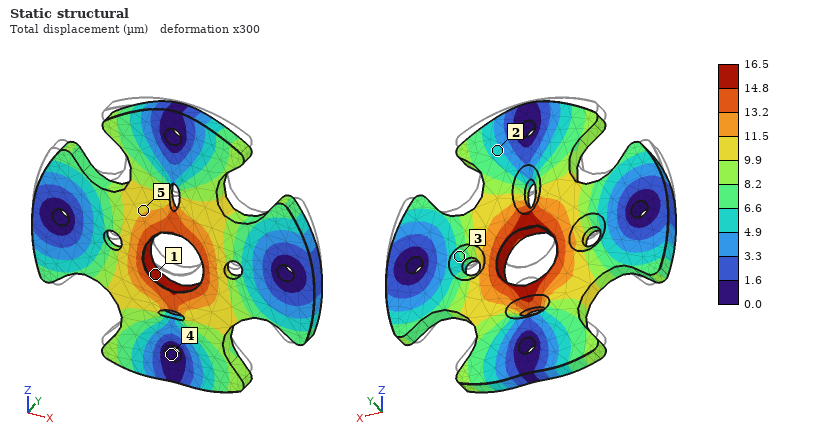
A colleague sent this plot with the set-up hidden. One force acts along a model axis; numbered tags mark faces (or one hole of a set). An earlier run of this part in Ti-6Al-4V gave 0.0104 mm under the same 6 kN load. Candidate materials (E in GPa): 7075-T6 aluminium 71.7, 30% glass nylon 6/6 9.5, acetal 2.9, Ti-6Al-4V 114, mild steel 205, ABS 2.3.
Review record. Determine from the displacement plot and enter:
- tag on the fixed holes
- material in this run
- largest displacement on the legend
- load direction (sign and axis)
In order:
4
7075-T6 aluminium
16.5 µm
-Z
